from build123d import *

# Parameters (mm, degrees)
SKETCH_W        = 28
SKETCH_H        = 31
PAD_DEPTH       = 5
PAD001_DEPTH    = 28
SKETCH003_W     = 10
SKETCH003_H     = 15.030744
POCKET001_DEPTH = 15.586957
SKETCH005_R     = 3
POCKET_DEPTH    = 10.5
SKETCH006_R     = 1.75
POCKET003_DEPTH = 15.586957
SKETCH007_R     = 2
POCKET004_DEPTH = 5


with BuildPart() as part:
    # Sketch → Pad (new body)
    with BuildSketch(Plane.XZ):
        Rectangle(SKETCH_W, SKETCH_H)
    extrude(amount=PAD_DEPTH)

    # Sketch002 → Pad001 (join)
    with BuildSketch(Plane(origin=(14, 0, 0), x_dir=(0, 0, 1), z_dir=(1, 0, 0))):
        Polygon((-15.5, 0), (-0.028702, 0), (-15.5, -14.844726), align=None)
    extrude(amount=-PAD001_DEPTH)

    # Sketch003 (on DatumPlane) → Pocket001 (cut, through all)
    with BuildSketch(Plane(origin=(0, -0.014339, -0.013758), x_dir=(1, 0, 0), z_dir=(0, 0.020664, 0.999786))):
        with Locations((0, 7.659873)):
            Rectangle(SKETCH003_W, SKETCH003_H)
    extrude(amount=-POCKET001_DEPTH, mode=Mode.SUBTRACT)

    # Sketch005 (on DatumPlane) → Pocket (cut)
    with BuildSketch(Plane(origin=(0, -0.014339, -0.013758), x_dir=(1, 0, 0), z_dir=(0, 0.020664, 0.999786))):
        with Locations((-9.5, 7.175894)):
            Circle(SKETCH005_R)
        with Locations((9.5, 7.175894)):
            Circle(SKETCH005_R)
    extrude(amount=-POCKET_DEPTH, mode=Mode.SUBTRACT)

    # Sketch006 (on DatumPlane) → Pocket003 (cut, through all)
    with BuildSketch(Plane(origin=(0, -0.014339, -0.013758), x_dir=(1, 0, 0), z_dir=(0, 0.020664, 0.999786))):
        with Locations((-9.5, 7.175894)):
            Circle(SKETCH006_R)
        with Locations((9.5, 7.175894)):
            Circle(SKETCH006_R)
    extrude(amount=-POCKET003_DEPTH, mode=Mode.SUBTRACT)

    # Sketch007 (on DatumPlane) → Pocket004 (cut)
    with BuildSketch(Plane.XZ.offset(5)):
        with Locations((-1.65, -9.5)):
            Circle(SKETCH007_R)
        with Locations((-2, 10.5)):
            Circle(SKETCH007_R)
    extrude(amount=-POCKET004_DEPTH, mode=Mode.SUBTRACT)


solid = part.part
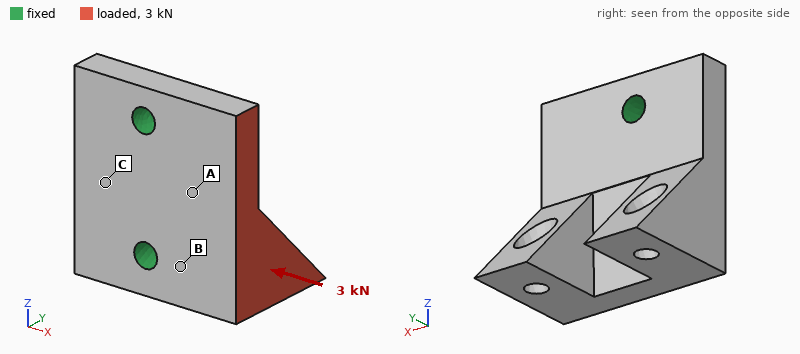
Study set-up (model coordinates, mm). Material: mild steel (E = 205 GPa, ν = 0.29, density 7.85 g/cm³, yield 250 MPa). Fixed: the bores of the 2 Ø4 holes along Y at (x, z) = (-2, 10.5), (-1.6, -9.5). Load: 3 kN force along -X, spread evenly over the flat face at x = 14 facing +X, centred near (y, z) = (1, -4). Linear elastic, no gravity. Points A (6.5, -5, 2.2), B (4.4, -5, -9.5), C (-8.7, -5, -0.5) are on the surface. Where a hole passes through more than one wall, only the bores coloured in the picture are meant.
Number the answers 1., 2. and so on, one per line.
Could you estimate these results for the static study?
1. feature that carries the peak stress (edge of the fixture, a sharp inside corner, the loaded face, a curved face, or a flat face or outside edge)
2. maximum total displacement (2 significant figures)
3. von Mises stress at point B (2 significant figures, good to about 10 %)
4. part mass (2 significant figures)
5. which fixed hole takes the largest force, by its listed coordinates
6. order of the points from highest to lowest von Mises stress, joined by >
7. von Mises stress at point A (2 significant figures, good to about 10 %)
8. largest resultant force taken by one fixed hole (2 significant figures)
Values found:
1. a flat face or outside edge
2. 45 µm
3. 70 MPa
4. 47 g
5. (-1.6, -9.5)
6. B > A > C
7. 47 MPa
8. 2.2 kN
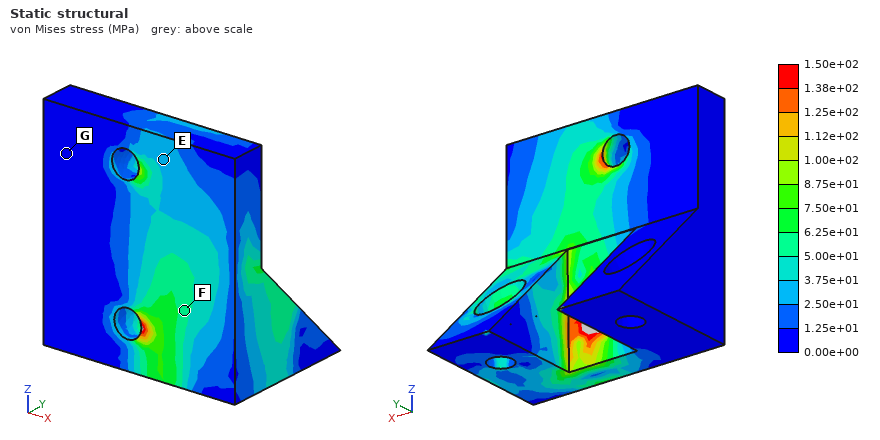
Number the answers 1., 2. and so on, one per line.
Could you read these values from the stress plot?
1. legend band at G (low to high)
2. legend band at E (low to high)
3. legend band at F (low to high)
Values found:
1. 0.00e+00 to 1.25e+01 MPa
2. 2.50e+01 to 3.75e+01 MPa
3. 5.00e+01 to 6.25e+01 MPa
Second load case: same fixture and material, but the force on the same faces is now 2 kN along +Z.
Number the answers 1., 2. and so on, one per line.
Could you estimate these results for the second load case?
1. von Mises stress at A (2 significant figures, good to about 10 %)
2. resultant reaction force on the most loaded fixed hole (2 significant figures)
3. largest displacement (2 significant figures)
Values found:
1. 26 MPa
2. 1.7 kN
3. 17 µm
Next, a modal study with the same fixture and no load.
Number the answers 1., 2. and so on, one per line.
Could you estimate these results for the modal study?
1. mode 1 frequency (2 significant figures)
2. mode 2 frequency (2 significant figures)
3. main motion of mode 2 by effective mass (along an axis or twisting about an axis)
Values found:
1. 9700 Hz
2. 14 kHz
3. along Y
